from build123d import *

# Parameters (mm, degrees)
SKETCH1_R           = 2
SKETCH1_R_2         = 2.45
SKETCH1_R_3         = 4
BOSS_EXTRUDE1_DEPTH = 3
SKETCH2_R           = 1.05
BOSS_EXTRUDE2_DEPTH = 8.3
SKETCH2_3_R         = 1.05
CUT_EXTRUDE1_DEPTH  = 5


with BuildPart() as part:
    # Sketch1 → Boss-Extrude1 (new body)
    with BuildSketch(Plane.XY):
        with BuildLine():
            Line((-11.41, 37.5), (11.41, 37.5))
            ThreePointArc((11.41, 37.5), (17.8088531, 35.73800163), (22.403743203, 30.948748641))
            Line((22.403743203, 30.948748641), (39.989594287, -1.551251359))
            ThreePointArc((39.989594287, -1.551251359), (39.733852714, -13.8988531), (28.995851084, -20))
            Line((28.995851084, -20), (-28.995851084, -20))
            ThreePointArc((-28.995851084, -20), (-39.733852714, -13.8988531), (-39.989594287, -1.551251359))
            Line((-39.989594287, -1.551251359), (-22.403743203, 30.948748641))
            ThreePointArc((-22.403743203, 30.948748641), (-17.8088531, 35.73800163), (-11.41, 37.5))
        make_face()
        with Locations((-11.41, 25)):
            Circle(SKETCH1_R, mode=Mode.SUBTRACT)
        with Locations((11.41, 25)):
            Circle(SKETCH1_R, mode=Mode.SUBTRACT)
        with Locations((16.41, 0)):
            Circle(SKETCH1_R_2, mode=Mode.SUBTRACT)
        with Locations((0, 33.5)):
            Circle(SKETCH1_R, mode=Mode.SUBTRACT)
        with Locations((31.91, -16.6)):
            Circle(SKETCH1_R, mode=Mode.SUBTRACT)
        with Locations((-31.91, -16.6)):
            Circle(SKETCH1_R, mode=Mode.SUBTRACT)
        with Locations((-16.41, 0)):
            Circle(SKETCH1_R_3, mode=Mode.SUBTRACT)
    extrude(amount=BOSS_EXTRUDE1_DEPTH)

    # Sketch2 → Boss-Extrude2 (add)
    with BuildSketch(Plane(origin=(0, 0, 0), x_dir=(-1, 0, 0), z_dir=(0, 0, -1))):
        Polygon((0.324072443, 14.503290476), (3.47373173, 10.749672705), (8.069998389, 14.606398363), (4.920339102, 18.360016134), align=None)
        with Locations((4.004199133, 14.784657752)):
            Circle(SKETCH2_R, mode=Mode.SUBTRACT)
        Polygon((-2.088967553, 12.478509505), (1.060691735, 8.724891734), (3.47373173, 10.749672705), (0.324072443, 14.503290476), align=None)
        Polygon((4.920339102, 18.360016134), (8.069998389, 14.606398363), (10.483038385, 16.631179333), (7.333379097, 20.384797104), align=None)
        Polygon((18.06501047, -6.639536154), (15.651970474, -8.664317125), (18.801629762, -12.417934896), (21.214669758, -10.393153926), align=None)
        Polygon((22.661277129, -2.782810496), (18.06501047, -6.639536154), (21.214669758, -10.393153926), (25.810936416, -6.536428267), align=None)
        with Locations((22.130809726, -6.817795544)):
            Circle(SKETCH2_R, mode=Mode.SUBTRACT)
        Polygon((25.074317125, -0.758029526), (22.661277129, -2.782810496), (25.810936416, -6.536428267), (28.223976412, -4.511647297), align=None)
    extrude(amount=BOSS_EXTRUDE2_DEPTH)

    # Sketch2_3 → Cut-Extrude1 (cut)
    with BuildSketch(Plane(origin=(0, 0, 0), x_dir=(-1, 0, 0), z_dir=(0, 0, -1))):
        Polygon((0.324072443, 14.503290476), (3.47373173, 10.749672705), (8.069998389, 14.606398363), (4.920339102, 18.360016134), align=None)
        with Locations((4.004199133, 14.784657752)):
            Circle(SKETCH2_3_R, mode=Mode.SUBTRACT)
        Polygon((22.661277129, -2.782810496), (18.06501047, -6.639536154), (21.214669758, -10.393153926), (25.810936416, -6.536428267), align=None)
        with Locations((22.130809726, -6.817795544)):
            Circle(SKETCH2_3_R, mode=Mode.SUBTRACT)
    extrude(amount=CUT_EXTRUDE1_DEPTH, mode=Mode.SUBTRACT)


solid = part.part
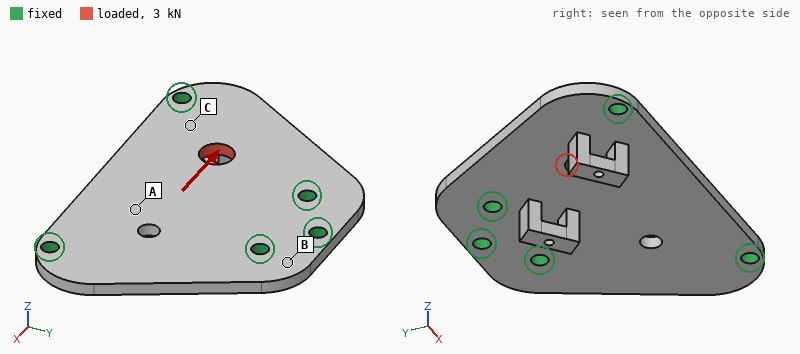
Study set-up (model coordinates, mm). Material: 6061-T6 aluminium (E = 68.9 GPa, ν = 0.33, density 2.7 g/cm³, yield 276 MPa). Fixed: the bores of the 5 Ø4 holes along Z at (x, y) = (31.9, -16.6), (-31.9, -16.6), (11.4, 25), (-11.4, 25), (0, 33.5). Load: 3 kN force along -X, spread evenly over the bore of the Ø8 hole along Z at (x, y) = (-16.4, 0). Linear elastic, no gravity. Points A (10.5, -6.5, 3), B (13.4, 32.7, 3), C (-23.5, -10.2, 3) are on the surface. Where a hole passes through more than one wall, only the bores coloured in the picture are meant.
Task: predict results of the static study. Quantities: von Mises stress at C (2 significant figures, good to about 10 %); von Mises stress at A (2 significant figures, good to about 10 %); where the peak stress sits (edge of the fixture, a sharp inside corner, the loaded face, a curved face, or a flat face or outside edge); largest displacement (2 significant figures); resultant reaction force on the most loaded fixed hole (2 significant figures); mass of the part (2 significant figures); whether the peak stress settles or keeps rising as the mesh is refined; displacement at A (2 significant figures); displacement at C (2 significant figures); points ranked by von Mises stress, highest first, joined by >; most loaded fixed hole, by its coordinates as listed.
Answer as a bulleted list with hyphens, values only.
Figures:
- 25 MPa
- 14 MPa
- edge of the fixture
- 15 µm
- 1.1 kN
- 31 g
- keeps rising
- 5.2 µm
- 7.1 µm
- C > A > B
- (-31.9, -16.6)
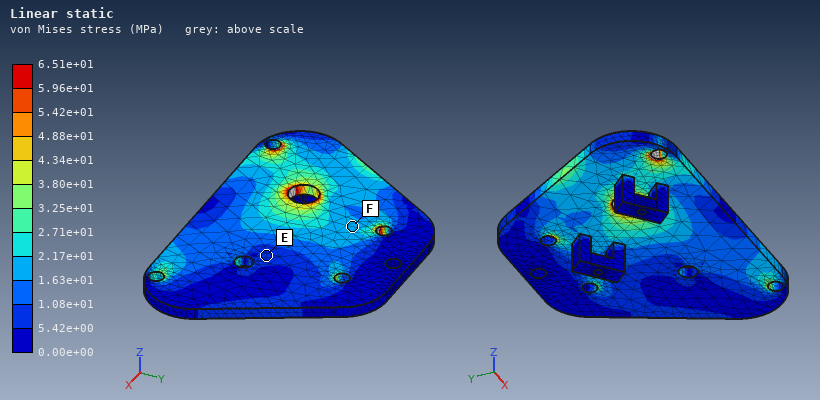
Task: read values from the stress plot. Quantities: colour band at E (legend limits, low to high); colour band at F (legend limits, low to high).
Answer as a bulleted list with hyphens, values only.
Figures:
- 5.42e+00 to 1.08e+01 MPa
- 1.63e+01 to 2.17e+01 MPa
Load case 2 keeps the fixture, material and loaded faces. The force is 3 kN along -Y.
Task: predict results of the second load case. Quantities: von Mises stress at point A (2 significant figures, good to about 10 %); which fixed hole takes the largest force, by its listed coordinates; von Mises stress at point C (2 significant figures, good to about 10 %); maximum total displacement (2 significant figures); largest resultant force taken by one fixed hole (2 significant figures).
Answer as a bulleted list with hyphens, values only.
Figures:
- 6.3 MPa
- (-11.4, 25)
- 28 MPa
- 14 µm
- 1.2 kN
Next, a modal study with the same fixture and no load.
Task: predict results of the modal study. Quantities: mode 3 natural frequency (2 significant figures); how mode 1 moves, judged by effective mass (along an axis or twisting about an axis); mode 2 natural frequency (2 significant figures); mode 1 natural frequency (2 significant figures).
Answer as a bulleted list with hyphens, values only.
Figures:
- 6600 Hz
- along Z
- 6400 Hz
- 4200 Hz
